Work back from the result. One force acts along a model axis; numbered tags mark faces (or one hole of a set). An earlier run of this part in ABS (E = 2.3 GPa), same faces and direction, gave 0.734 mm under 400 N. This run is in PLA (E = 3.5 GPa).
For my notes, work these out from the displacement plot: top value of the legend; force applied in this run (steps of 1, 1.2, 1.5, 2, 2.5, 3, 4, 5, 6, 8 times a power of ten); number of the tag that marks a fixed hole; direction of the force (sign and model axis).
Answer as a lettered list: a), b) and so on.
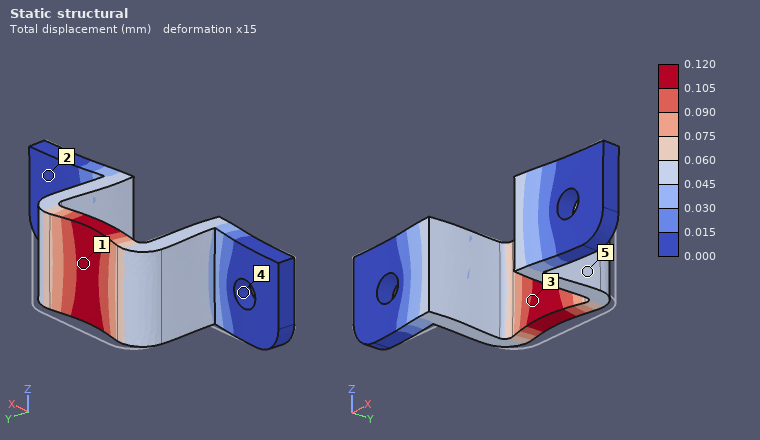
a) 0.120 mm
b) 100 N
c) 4
d) -Y
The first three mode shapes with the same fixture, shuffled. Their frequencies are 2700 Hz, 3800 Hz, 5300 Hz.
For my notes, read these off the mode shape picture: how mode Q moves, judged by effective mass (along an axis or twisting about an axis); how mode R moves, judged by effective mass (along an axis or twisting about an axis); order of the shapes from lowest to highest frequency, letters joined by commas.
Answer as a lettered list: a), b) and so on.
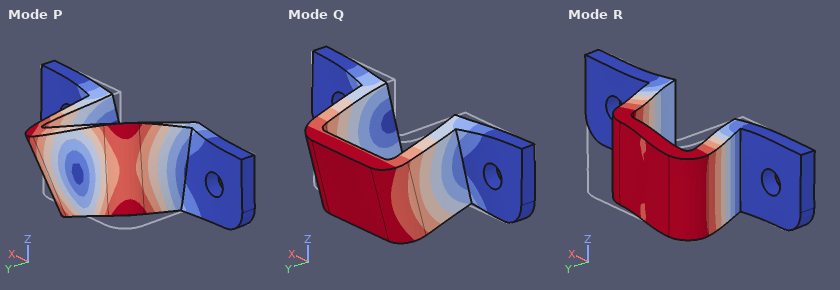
a) along Z
b) along X
c) Q, R, P
